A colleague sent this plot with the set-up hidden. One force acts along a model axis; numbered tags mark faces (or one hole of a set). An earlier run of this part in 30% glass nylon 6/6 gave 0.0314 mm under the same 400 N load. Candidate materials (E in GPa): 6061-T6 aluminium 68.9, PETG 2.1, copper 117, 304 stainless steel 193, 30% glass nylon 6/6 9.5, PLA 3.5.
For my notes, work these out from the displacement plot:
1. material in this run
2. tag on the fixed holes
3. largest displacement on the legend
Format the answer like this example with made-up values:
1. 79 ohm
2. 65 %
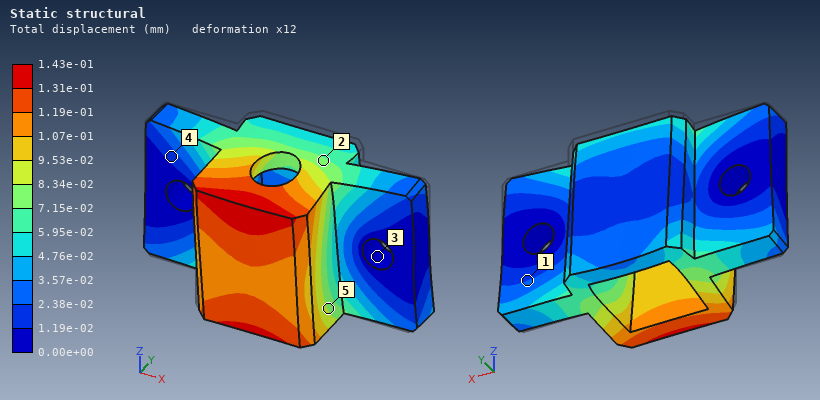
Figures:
1. PETG
2. 3
3. 1.43e-01 mm
